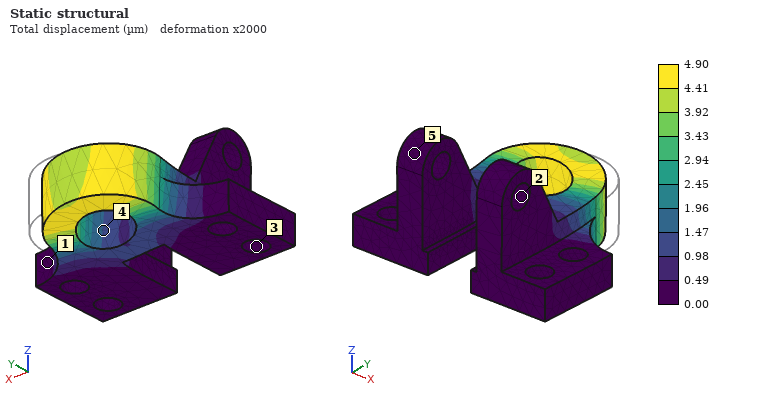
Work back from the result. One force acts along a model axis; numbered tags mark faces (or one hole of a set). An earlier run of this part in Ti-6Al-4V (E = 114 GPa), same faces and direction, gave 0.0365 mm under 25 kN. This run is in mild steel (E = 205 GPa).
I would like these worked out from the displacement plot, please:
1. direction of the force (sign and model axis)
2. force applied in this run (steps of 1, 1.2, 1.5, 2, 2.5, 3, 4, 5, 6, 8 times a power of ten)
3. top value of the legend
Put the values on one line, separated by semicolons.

-X; 6 kN; 4.90 µm
